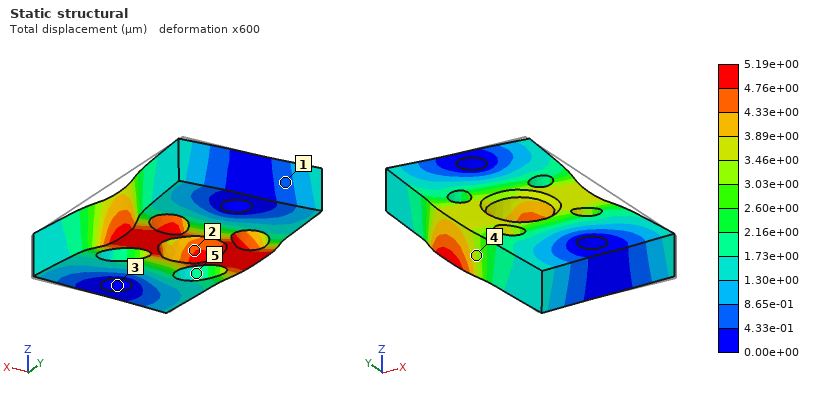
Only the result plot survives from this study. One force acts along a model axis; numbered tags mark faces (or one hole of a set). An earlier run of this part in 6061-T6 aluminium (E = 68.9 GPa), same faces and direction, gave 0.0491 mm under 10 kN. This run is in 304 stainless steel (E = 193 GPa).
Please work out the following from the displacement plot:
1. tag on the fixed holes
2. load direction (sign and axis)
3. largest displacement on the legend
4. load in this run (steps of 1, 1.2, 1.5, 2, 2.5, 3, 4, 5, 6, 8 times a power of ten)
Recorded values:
3
-X
5.19e+00 µm
3 kN
